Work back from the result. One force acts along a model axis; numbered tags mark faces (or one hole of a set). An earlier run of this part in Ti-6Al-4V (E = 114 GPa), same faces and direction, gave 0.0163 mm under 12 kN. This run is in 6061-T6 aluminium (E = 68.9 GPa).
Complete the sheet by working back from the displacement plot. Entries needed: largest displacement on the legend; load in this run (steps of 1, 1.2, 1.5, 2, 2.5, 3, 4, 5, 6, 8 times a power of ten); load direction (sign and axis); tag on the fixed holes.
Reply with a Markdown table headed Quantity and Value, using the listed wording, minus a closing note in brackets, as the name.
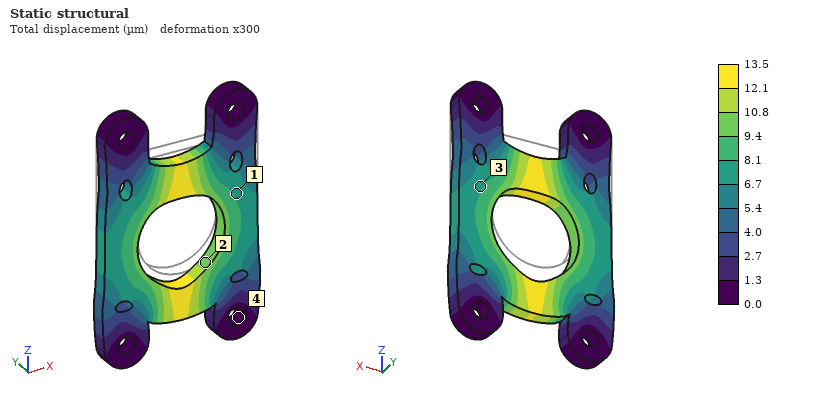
| Quantity | Value |
|---|---|
| largest displacement on the legend | 13.5 µm |
| load in this run | 6 kN |
| load direction | -Z |
| tag on the fixed holes | 4 |
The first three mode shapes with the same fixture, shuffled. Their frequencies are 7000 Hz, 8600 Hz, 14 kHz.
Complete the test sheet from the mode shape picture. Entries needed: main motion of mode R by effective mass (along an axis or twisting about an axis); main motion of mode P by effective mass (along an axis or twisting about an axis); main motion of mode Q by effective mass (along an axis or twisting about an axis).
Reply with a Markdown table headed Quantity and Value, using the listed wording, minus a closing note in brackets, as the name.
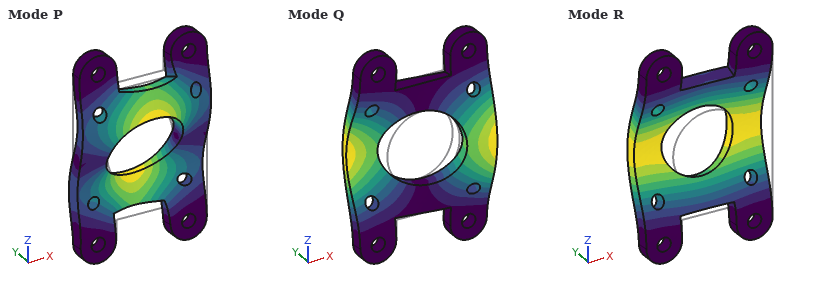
| Quantity | Value |
|---|---|
| main motion of mode R by effective mass | along Y |
| main motion of mode P by effective mass | twisting about X |
| main motion of mode Q by effective mass | twisting about Z |
